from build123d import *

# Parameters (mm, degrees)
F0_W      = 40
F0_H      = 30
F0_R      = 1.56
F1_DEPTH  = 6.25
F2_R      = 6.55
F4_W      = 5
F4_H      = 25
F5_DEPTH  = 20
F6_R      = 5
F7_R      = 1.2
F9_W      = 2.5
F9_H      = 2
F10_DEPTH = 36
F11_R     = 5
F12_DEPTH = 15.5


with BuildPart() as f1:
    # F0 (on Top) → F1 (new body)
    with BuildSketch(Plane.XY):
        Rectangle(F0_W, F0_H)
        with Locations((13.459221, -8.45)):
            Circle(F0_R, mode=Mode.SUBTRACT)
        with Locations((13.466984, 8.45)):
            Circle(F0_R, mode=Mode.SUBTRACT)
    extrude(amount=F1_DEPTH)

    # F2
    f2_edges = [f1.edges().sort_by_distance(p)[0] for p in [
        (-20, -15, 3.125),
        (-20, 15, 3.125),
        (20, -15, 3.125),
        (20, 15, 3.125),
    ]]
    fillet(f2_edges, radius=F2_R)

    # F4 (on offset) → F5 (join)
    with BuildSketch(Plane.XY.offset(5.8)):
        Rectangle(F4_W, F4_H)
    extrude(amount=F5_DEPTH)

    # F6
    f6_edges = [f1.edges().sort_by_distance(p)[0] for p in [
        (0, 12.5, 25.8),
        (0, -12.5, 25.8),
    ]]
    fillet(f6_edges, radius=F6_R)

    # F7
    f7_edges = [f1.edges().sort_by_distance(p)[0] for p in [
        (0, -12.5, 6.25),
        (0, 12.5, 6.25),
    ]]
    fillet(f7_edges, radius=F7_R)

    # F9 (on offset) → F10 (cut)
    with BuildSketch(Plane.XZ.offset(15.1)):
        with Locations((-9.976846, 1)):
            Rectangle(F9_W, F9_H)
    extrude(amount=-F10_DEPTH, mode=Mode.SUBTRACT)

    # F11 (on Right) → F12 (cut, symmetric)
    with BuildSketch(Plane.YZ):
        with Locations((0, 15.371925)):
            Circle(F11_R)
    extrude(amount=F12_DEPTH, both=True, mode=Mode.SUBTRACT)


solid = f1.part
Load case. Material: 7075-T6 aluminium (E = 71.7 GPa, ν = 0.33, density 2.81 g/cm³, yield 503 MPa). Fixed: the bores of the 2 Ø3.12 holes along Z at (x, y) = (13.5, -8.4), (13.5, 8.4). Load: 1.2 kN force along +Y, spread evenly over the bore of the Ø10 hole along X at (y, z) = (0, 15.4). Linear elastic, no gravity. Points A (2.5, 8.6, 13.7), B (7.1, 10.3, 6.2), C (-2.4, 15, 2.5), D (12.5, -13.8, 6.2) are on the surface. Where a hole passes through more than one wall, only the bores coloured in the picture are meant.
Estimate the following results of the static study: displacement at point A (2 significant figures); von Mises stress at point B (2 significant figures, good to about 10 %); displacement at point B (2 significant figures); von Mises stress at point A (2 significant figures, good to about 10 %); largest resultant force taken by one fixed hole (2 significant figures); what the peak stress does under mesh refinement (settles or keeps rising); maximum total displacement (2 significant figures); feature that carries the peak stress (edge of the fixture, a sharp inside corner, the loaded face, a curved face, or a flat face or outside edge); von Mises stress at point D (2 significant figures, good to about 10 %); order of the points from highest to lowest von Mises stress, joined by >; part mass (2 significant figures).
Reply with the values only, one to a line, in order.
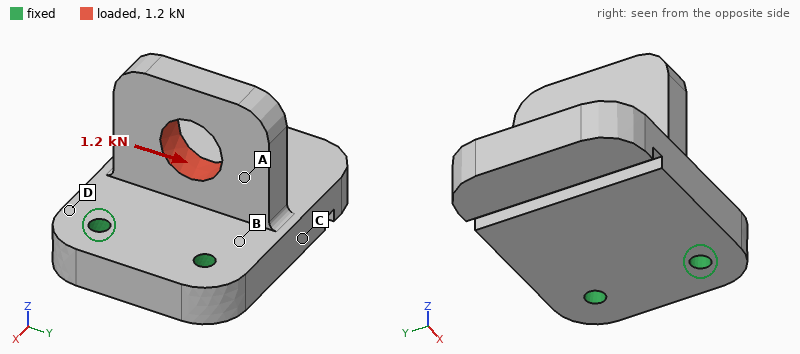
29 µm
38 MPa
8.4 µm
29 MPa
1.2 kN
keeps rising
52 µm
edge of the fixture
19 MPa
B > A > D > C
25 g
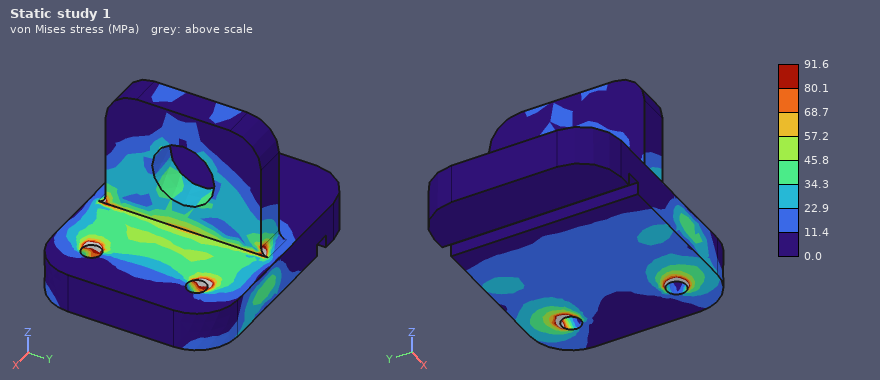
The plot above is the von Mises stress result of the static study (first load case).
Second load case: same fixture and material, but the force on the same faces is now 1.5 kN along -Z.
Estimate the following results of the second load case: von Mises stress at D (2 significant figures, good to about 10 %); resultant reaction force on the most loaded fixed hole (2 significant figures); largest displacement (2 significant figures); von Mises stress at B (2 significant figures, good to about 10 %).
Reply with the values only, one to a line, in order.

46 MPa
750 N
0.11 mm
56 MPa
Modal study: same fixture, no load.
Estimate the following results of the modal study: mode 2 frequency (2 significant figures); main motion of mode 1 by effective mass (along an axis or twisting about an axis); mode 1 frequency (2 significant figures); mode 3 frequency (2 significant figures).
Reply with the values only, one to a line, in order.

8700 Hz
along Z
3800 Hz
9300 Hz
